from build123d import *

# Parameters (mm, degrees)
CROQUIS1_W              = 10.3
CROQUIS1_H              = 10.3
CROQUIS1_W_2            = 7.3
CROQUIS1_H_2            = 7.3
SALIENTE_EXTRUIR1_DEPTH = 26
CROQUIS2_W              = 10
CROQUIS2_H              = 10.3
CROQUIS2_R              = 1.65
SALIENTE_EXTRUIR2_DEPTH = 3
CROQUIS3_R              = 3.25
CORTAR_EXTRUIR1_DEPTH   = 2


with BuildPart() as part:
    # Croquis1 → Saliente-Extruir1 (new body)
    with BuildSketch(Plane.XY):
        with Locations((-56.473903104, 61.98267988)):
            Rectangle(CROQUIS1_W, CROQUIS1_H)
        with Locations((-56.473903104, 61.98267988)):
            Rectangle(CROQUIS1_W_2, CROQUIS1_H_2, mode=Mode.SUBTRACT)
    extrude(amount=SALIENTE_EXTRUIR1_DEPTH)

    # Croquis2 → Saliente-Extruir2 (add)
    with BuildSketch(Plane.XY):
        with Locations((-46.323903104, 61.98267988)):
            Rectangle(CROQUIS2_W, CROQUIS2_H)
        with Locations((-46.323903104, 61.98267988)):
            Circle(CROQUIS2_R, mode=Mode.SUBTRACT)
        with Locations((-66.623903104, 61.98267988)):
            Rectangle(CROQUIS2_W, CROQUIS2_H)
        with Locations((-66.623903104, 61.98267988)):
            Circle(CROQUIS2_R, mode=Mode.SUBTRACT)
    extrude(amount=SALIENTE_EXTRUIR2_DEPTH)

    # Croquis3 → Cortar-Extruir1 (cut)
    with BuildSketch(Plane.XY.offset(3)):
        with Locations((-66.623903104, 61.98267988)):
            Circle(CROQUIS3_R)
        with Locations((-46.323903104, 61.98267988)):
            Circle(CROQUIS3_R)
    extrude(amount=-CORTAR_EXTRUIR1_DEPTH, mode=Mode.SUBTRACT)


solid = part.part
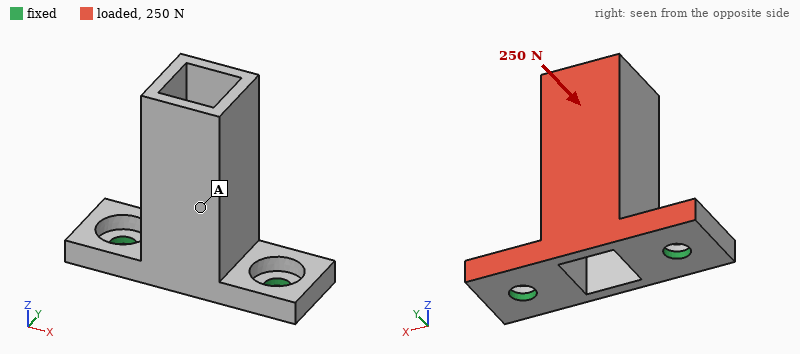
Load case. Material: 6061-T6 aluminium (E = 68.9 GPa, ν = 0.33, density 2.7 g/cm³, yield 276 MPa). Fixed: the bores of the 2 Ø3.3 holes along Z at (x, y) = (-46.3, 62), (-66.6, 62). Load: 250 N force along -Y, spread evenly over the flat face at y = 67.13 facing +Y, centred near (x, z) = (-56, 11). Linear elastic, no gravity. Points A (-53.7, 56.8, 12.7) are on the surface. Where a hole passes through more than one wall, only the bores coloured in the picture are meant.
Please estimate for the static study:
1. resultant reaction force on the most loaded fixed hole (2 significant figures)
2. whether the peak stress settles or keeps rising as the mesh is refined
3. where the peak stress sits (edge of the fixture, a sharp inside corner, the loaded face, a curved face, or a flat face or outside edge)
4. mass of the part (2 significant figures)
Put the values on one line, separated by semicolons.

130 N; keeps rising; edge of the fixture; 5.0 g
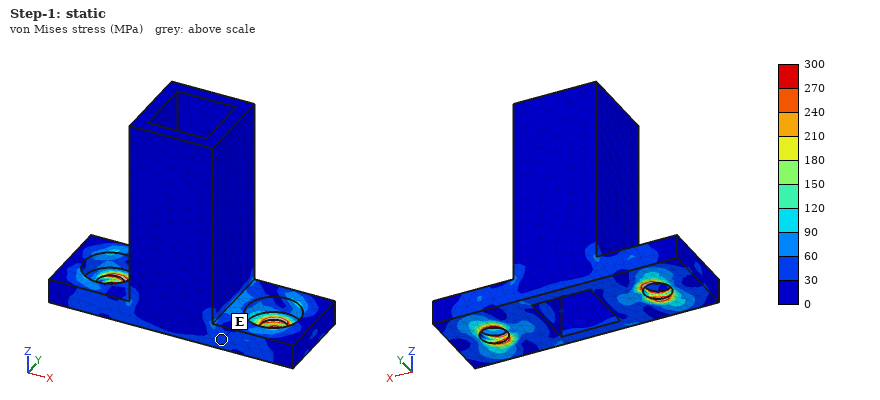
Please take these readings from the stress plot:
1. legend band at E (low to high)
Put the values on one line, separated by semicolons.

30 to 60 MPa
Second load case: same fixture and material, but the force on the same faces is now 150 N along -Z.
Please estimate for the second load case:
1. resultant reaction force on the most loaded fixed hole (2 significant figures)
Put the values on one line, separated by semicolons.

95 N
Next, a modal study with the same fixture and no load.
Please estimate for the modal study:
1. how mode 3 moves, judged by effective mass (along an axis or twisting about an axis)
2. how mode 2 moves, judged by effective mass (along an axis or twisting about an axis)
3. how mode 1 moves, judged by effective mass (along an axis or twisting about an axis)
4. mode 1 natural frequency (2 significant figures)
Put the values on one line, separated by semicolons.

along Z; along X; along Y; 3000 Hz
